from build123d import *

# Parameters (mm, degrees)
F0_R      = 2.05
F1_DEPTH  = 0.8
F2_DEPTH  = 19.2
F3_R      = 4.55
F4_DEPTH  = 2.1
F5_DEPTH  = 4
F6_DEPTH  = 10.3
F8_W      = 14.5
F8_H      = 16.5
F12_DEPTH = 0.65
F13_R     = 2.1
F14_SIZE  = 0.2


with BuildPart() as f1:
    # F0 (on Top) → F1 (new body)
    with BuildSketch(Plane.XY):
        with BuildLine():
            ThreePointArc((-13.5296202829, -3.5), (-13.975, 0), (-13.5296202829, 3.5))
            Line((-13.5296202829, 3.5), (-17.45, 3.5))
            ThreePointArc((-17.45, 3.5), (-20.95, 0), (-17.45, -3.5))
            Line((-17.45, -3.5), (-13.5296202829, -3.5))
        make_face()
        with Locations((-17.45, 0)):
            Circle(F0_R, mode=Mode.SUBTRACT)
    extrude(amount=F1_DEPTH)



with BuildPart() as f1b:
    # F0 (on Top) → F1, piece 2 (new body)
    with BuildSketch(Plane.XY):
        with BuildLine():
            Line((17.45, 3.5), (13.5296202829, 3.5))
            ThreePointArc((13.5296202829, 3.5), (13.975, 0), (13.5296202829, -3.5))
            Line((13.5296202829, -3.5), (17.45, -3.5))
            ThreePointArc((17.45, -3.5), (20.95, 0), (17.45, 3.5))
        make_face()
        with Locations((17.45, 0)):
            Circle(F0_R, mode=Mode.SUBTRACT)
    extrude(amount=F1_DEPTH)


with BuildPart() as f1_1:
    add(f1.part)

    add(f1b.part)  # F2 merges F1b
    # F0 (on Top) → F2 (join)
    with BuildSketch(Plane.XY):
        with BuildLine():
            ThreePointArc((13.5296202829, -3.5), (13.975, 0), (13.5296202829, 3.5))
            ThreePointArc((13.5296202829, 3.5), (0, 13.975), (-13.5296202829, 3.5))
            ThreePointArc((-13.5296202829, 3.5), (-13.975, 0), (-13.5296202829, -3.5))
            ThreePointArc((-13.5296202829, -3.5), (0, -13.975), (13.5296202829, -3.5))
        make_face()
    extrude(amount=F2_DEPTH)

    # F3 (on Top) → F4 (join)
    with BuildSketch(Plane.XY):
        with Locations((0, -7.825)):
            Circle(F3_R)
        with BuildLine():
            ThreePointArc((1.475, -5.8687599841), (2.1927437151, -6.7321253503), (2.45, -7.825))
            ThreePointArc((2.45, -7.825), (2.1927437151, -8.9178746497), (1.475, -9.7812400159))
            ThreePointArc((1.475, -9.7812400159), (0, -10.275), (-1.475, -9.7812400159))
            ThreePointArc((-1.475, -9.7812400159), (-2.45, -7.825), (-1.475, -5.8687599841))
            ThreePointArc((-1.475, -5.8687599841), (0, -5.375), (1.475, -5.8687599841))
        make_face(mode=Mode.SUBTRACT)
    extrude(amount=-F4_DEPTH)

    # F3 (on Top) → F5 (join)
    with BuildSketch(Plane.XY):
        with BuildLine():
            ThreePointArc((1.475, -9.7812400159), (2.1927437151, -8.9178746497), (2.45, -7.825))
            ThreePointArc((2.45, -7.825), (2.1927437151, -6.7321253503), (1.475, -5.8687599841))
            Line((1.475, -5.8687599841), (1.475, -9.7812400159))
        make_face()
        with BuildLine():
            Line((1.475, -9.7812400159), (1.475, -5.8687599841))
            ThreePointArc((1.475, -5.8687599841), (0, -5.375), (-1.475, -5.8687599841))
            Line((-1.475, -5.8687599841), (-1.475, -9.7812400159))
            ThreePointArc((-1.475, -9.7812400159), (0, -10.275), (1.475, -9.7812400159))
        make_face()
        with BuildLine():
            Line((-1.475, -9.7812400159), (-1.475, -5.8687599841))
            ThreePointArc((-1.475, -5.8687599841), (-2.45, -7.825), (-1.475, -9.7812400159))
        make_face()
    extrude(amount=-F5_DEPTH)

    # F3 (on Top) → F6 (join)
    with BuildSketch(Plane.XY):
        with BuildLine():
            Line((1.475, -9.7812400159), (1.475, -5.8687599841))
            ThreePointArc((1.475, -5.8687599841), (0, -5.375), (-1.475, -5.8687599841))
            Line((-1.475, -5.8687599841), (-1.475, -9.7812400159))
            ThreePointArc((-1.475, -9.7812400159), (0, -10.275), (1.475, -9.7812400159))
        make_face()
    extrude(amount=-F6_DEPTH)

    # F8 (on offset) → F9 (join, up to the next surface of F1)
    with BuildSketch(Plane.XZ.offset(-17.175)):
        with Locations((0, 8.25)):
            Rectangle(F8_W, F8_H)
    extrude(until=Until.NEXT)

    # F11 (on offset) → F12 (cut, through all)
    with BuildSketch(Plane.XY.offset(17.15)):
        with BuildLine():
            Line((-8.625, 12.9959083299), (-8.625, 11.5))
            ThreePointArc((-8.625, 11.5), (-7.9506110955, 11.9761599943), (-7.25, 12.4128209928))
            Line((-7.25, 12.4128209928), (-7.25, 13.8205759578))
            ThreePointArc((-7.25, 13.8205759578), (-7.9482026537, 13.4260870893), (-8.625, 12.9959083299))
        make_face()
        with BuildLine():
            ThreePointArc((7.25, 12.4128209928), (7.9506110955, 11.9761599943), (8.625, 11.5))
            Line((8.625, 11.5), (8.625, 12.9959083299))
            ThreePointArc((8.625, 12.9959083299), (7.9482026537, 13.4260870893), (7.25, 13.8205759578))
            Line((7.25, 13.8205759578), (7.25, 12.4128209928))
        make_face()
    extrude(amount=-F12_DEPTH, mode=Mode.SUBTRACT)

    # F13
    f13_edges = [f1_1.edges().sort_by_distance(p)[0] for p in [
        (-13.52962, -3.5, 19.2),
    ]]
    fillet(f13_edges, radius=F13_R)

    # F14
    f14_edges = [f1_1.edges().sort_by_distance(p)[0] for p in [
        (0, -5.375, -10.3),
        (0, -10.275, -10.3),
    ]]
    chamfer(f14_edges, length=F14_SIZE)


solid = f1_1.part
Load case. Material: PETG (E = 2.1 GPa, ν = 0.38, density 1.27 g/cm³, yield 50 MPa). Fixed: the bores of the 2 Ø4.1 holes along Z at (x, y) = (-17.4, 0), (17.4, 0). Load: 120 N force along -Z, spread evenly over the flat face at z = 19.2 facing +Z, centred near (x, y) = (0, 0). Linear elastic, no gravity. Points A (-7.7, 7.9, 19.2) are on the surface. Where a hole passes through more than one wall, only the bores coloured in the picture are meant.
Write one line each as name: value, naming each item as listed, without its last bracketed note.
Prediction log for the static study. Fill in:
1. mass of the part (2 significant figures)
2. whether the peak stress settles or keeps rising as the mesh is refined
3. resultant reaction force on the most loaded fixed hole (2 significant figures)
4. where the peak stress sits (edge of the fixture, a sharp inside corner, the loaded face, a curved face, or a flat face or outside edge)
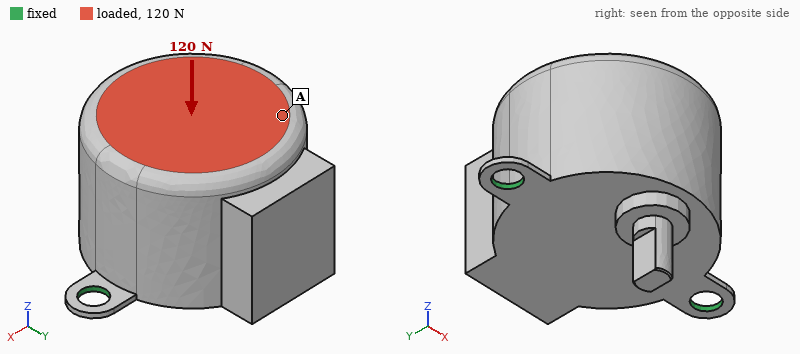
mass of the part: 16 g
whether the peak stress settles or keeps rising as the mesh is refined: keeps rising
resultant reaction force on the most loaded fixed hole: 71 N
where the peak stress sits: edge of the fixture
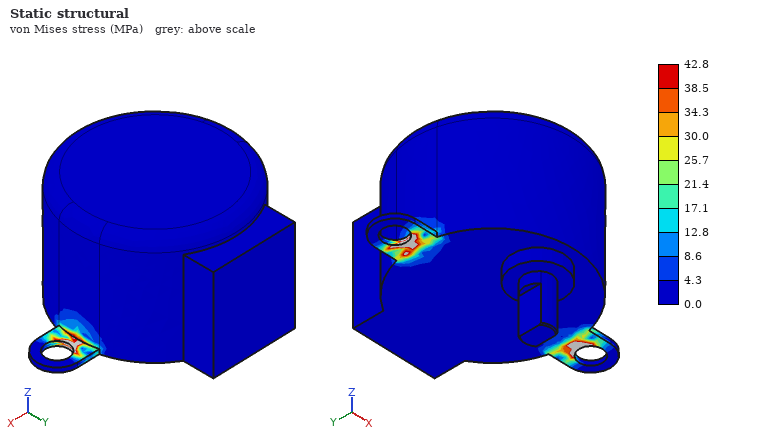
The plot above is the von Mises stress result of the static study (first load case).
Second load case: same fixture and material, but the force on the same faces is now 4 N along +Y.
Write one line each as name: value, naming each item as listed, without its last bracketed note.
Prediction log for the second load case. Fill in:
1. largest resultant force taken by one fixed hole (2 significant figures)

largest resultant force taken by one fixed hole: 2.0 N
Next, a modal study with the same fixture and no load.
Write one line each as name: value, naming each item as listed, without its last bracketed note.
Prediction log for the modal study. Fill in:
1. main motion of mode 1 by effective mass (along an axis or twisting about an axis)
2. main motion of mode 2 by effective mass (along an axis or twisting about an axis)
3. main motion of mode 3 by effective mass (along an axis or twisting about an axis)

main motion of mode 1 by effective mass: along Y
main motion of mode 2 by effective mass: along Z
main motion of mode 3 by effective mass: along X
